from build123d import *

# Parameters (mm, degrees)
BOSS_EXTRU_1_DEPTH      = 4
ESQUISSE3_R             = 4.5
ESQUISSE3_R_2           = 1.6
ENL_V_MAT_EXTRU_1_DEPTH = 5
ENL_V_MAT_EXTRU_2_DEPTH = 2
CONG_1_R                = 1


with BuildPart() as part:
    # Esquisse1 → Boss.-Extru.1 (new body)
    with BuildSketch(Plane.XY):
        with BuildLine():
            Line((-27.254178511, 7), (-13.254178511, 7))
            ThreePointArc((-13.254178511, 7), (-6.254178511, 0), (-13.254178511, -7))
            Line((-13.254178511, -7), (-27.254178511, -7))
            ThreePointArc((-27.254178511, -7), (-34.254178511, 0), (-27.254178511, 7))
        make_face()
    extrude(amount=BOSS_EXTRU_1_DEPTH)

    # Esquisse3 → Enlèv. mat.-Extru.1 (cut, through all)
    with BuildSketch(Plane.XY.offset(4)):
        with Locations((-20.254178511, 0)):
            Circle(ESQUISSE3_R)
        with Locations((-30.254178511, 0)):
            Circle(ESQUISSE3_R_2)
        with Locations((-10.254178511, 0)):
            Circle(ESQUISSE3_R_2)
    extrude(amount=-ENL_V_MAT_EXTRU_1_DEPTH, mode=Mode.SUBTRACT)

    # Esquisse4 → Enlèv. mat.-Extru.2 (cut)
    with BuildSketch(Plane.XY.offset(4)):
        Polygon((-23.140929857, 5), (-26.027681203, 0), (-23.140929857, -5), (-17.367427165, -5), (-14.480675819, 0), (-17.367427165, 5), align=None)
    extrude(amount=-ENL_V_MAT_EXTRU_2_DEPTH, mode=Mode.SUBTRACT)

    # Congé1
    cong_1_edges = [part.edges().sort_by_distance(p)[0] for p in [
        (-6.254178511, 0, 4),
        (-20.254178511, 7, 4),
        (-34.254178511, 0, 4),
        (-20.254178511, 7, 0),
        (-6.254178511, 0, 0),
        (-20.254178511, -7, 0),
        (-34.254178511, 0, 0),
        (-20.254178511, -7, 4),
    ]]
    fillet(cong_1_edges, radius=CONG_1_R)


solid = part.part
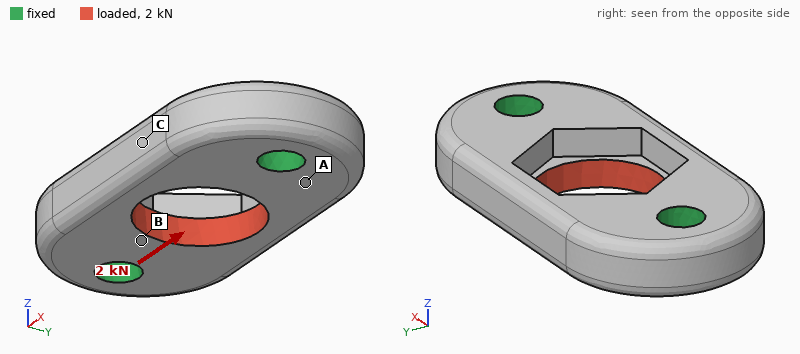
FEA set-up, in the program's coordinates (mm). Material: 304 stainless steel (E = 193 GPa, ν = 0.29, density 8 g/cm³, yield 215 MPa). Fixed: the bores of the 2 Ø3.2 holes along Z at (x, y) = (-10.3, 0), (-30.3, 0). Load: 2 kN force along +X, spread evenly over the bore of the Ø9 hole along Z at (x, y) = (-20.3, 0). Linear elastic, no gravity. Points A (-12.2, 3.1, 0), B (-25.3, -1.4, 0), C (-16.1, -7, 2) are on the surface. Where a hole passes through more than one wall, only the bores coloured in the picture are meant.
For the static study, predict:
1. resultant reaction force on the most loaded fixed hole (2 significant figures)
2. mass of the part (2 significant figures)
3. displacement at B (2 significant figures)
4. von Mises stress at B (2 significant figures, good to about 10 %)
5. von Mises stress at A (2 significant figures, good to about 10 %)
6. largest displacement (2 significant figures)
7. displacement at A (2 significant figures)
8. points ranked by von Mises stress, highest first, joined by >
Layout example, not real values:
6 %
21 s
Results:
1.0 kN
8.0 g
1.1 µm
57 MPa
30 MPa
2.1 µm
0.70 µm
B > A > C
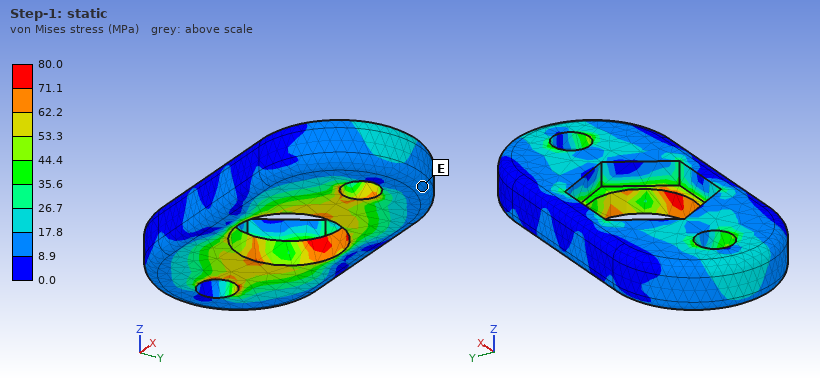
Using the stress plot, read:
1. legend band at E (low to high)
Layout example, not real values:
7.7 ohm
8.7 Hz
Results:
8.9 to 17.8 MPa
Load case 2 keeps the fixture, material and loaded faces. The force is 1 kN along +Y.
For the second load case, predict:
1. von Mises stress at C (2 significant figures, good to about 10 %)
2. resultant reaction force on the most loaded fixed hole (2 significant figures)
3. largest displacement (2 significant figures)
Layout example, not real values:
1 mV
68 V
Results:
18 MPa
500 N
3.0 µm
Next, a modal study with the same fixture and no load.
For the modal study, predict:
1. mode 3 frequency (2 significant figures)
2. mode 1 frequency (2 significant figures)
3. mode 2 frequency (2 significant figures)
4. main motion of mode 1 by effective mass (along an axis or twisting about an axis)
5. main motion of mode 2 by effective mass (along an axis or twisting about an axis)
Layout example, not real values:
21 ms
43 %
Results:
61 kHz
40 kHz
42 kHz
twisting about X
along Z
